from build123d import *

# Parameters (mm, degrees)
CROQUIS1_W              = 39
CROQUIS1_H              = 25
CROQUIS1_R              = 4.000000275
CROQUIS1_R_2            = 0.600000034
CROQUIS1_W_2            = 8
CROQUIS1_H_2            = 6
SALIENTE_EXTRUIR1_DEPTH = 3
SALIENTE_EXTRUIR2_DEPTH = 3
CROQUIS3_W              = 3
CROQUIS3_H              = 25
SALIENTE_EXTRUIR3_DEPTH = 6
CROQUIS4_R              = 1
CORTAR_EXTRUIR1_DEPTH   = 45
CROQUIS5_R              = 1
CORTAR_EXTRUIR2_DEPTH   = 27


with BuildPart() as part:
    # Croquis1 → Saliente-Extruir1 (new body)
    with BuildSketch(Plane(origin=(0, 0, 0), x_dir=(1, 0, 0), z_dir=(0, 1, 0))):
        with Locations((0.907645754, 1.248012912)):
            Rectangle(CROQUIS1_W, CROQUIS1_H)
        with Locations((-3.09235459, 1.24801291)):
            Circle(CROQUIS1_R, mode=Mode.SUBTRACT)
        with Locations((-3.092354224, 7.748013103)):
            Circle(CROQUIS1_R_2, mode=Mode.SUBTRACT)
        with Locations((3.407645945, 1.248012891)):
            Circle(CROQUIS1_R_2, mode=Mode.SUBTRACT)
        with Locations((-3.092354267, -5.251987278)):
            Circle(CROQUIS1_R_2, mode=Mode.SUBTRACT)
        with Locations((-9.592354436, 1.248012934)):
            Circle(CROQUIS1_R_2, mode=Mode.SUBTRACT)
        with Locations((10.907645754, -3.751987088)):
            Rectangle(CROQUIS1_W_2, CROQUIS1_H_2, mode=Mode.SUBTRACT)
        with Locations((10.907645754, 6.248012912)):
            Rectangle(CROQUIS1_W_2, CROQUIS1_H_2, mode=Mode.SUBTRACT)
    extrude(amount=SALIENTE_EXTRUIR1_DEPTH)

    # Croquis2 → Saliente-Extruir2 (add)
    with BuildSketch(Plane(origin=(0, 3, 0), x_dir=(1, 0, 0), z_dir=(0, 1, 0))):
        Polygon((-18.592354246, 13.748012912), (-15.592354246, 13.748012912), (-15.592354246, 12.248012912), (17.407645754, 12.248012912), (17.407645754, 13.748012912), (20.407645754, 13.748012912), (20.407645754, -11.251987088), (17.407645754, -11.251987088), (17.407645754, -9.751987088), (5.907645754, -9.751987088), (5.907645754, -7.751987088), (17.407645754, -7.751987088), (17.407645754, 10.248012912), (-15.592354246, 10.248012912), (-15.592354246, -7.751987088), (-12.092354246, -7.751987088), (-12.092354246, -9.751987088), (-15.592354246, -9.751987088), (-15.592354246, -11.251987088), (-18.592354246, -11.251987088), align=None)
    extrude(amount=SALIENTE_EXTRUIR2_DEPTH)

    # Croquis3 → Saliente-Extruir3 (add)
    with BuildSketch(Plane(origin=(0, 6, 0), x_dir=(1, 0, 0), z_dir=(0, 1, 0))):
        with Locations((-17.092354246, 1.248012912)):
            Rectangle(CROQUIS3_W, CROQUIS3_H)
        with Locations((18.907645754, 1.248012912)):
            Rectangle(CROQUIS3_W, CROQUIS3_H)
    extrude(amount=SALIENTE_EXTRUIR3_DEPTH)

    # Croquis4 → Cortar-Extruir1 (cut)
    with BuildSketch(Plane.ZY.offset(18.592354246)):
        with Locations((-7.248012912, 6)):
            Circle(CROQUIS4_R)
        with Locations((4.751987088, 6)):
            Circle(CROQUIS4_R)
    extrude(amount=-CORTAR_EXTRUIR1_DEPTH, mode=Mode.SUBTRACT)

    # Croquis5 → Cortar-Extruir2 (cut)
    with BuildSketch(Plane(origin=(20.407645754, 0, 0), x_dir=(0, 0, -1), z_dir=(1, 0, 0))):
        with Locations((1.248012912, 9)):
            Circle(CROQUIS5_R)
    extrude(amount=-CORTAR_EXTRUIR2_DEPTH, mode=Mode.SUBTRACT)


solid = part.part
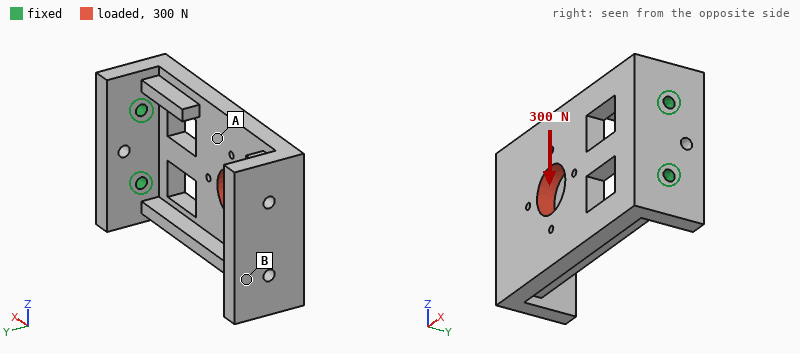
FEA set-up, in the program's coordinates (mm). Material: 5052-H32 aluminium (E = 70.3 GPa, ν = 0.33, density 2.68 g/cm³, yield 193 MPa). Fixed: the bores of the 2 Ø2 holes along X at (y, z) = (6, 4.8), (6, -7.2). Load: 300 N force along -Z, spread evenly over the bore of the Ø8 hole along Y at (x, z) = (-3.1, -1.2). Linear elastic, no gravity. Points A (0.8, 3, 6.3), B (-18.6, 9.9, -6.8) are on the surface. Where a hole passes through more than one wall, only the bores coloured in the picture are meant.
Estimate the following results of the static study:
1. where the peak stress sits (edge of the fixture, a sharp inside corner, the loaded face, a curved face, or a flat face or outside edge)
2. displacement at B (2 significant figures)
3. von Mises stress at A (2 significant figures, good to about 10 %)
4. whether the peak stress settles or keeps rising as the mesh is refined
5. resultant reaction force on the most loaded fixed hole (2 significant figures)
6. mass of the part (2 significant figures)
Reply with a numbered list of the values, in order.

1. edge of the fixture
2. 0.091 mm
3. 19 MPa
4. keeps rising
5. 460 N
6. 11 g
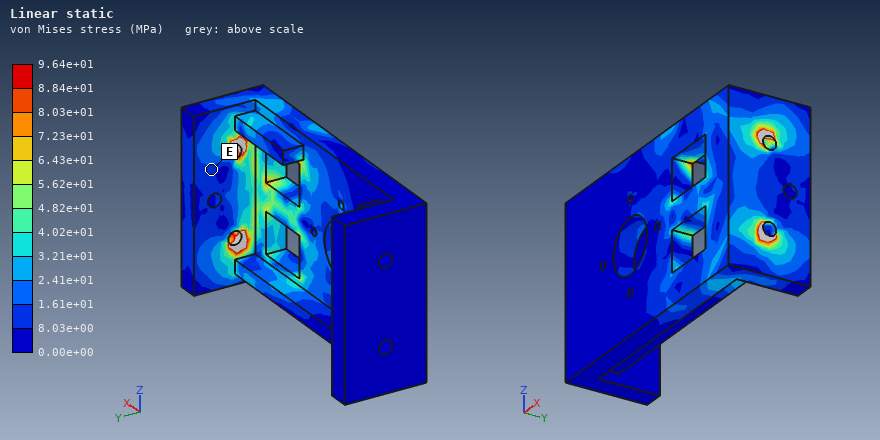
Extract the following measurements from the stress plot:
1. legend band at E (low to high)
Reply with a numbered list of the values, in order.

1. 8.03e+00 to 1.61e+01 MPa
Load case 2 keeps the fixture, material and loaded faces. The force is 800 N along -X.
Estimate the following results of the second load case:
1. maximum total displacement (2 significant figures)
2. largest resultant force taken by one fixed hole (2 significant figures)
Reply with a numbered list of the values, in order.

1. 0.12 mm
2. 400 N
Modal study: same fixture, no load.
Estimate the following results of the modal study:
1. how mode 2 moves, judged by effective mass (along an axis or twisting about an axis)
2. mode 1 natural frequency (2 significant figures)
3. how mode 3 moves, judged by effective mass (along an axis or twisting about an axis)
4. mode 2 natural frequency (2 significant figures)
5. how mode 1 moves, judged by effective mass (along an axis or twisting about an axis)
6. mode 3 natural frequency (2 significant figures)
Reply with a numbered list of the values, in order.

1. along Z
2. 1400 Hz
3. along Z
4. 2900 Hz
5. along Y
6. 5400 Hz
